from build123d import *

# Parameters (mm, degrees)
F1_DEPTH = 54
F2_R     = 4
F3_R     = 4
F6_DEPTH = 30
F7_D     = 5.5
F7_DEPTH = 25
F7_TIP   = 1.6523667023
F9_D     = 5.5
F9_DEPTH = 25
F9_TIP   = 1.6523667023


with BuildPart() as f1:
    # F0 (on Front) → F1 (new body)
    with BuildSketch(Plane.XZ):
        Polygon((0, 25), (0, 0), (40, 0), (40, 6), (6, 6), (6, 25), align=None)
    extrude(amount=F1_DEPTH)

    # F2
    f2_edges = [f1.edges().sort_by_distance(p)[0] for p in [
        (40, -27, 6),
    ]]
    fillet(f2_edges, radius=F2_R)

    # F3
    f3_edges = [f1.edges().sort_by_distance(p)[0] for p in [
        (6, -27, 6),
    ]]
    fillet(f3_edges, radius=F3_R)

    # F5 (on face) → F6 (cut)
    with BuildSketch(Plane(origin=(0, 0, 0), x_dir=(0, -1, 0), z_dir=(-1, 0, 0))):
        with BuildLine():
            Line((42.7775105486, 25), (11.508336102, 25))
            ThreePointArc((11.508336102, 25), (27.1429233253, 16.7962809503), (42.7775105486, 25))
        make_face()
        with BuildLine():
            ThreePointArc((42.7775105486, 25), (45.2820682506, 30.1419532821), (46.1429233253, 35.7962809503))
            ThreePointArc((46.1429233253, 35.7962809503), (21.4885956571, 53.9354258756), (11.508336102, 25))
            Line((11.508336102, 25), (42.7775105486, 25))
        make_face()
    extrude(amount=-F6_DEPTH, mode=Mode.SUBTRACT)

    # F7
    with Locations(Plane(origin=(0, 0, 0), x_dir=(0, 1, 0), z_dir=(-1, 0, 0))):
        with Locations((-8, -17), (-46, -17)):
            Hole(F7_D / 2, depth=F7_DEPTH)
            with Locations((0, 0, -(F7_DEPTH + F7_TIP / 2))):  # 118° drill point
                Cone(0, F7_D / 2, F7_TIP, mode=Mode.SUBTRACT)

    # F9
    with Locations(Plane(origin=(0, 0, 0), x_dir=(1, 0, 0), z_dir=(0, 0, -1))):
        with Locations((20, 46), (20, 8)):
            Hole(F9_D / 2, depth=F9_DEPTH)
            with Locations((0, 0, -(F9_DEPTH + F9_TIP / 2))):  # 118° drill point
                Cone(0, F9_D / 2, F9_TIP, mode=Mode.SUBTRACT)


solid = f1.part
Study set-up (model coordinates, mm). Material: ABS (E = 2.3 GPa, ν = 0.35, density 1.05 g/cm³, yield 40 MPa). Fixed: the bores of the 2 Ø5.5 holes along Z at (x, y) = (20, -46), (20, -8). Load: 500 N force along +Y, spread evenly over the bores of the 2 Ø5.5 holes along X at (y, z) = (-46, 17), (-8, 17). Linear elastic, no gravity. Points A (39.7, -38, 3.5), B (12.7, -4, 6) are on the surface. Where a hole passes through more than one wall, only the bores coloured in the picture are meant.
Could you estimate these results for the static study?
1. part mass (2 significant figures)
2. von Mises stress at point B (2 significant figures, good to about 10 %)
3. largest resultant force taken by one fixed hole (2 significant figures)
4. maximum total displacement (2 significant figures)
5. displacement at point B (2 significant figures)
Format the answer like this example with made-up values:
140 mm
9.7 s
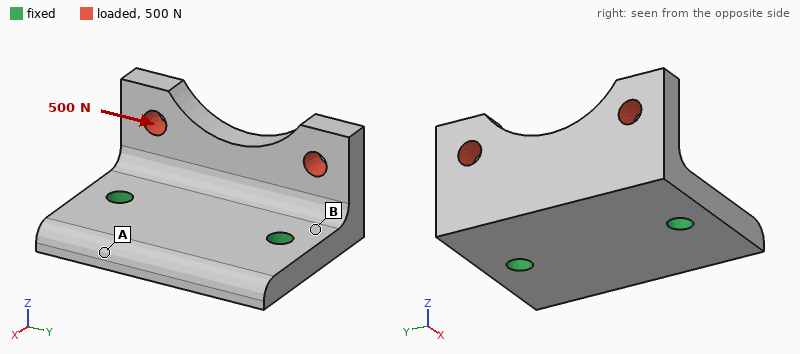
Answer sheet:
18 g
7.6 MPa
360 N
0.39 mm
0.068 mm
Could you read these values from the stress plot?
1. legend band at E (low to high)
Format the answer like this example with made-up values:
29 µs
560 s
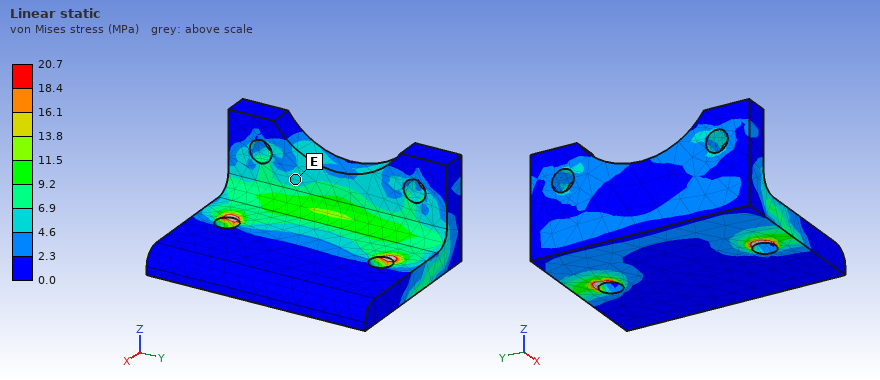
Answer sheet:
4.6 to 6.9 MPa
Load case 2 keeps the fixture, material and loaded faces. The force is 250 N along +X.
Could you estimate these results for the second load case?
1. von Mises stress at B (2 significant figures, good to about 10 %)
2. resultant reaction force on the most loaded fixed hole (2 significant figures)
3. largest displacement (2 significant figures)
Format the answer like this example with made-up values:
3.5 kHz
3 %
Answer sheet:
13 MPa
130 N
0.73 mm
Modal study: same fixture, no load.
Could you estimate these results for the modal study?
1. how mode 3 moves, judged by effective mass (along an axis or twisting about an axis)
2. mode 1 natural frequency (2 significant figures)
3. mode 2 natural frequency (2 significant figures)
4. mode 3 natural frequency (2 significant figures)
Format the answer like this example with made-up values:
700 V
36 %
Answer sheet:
along Z
1500 Hz
2300 Hz
3200 Hz
